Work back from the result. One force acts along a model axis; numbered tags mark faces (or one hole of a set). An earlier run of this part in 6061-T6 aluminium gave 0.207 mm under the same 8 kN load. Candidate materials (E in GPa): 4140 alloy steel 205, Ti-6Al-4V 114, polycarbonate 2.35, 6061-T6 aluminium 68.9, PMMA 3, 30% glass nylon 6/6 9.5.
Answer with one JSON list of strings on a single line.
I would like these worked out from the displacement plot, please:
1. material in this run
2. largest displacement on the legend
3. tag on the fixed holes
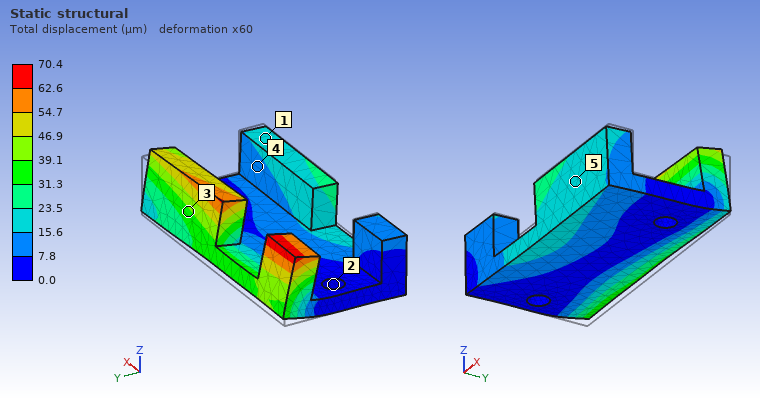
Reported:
["4140 alloy steel", "70.4 µm", "2"]
